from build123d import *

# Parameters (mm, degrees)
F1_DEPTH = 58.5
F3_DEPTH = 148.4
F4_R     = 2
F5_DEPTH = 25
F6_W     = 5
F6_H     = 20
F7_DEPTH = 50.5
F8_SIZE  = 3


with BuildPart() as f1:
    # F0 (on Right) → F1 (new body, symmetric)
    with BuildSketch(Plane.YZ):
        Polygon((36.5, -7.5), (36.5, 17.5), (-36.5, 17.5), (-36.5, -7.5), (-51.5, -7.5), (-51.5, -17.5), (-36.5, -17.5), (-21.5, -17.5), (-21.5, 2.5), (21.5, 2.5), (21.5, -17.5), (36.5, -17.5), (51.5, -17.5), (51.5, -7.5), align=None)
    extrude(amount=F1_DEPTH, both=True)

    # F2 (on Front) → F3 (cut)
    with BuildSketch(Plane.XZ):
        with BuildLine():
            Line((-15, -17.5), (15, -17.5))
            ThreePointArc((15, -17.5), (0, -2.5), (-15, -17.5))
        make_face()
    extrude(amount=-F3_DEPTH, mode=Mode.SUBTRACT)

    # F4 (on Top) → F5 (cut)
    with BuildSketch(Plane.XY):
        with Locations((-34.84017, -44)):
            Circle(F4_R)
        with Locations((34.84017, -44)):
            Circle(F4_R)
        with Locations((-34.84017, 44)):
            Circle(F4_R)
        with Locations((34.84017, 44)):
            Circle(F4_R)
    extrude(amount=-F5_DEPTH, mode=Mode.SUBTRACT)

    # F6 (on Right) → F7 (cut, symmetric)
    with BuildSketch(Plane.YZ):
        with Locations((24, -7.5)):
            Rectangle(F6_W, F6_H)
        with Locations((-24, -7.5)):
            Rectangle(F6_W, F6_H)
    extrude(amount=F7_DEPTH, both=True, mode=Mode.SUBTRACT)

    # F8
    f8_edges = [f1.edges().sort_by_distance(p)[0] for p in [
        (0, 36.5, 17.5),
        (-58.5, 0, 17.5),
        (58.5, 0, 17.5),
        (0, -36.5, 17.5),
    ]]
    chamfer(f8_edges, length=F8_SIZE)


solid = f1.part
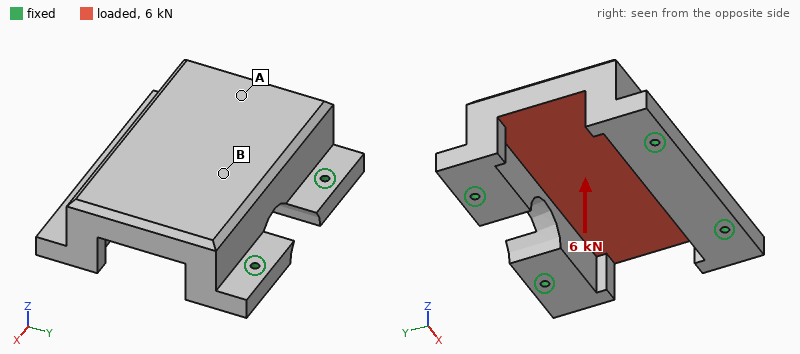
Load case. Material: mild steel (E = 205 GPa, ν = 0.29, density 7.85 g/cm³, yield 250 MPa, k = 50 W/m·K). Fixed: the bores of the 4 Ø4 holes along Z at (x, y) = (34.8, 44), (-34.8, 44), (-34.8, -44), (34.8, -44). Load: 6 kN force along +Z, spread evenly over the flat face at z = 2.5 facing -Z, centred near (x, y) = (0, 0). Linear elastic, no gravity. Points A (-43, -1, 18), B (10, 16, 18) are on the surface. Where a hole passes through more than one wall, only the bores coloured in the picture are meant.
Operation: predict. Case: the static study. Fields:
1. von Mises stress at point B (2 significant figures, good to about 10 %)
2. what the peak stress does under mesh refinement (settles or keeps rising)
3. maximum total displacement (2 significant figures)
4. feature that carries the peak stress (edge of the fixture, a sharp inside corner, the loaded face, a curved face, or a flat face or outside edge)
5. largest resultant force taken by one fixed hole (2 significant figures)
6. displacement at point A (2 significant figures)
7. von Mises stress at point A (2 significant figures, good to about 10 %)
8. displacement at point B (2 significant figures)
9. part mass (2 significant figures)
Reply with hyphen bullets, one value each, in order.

- 3.8 MPa
- keeps rising
- 4.0 µm
- edge of the fixture
- 1.9 kN
- 3.5 µm
- 7.1 MPa
- 3.4 µm
- 1.6 kg
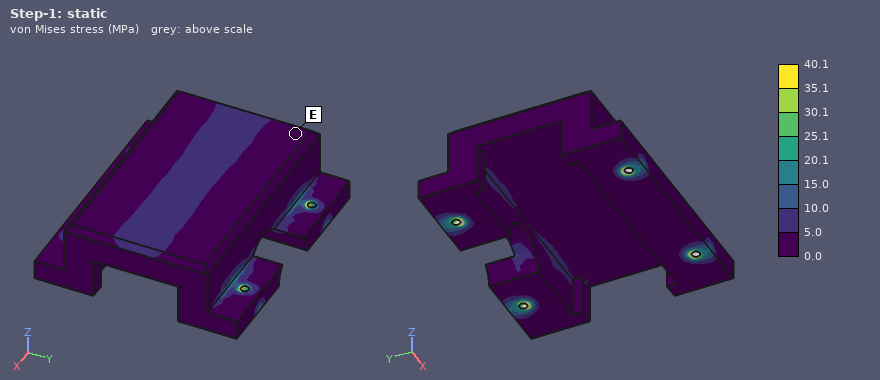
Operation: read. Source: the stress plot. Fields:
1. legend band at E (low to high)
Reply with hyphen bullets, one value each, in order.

- 0.0 to 5.0 MPa
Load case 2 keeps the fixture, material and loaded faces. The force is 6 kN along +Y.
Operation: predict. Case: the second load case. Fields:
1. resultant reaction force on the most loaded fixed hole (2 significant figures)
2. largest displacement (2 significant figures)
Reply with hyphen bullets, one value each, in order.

- 1.6 kN
- 3.9 µm
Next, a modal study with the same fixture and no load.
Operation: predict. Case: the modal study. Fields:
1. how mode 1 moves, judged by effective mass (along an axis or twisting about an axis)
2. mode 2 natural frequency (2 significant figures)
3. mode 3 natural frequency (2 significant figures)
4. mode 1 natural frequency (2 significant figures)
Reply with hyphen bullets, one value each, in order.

- along X
- 6400 Hz
- 6500 Hz
- 5400 Hz
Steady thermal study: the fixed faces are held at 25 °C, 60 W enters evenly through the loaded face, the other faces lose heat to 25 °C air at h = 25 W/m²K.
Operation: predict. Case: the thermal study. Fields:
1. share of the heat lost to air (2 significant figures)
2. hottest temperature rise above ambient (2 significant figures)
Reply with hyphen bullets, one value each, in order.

- 20 %
- 25 K
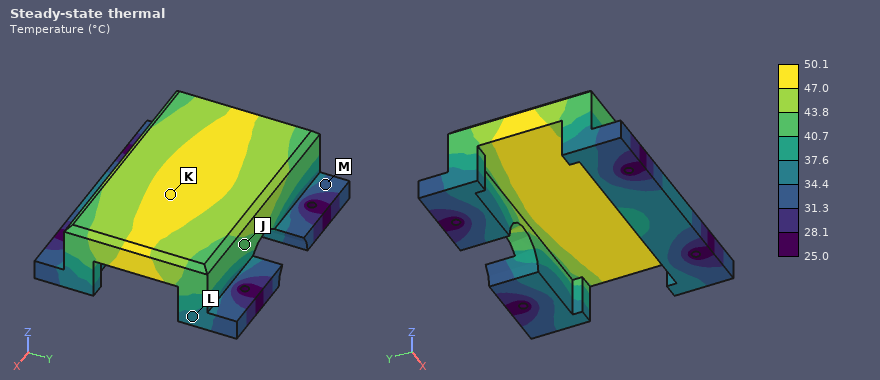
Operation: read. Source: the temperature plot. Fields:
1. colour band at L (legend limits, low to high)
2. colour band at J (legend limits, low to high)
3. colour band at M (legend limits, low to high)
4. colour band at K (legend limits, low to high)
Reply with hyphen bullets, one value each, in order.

- 34.4 to 37.6 °C
- 40.7 to 43.8 °C
- 31.3 to 34.4 °C
- 47.0 to 50.1 °C
